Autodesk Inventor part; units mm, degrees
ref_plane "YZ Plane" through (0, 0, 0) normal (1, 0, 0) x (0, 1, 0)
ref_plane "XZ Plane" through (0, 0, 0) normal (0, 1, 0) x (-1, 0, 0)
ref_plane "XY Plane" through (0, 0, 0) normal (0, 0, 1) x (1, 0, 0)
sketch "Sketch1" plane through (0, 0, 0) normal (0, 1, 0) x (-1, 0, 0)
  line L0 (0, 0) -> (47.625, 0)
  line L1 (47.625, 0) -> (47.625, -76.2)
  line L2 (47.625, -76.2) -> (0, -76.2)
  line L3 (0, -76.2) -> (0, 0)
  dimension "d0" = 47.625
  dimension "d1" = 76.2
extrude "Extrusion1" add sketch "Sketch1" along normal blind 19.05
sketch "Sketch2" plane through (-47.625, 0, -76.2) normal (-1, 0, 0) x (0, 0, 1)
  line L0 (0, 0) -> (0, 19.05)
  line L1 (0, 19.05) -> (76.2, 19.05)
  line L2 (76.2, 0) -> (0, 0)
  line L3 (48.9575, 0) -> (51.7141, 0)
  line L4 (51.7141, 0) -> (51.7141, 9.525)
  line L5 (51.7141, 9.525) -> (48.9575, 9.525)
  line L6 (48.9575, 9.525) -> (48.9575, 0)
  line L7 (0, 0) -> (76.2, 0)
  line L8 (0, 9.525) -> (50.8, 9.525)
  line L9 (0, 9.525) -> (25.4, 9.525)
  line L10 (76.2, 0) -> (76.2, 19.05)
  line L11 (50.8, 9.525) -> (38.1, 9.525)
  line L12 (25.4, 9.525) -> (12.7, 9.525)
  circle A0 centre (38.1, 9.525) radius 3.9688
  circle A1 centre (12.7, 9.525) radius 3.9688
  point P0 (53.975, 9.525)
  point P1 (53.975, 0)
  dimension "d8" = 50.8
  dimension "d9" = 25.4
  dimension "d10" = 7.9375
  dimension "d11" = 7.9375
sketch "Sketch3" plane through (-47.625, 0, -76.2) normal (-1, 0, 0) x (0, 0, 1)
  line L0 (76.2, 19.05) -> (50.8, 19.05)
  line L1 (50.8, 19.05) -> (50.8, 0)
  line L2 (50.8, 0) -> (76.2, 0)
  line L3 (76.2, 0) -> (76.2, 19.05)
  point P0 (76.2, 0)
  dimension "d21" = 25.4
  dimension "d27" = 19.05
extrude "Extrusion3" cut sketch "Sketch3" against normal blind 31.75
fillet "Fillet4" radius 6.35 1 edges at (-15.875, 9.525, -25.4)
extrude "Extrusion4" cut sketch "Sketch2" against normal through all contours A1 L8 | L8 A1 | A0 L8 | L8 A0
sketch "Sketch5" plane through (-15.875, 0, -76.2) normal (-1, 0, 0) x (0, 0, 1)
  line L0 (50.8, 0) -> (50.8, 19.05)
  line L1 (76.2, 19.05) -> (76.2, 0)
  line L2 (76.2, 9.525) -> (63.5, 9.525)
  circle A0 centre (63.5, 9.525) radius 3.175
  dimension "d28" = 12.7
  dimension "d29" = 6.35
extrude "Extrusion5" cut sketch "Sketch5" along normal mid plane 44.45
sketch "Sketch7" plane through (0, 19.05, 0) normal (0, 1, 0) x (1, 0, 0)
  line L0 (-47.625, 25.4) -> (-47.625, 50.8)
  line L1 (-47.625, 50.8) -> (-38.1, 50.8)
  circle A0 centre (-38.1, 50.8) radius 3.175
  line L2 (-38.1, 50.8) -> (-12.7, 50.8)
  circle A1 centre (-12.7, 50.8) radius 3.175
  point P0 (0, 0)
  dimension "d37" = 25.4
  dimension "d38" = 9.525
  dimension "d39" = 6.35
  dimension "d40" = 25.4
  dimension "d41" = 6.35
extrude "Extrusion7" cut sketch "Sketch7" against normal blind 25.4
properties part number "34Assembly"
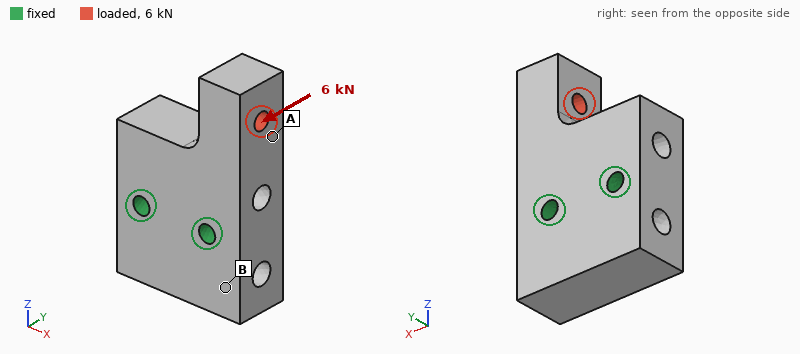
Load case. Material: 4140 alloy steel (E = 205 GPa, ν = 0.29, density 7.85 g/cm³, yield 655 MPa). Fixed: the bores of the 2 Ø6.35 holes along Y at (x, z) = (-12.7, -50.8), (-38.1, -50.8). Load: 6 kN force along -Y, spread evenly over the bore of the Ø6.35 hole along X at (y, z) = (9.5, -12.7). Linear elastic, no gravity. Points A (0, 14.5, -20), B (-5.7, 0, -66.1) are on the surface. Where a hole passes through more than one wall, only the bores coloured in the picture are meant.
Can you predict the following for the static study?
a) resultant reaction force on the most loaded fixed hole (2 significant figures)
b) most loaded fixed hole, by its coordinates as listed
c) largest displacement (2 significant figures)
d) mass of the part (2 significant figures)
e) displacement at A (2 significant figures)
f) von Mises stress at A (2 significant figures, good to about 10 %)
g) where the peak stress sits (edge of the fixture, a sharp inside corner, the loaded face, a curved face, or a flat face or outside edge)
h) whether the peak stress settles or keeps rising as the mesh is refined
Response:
5.4 kN
(-12.7, -50.8)
70 µm
370 g
36 µm
37 MPa
edge of the fixture
keeps rising
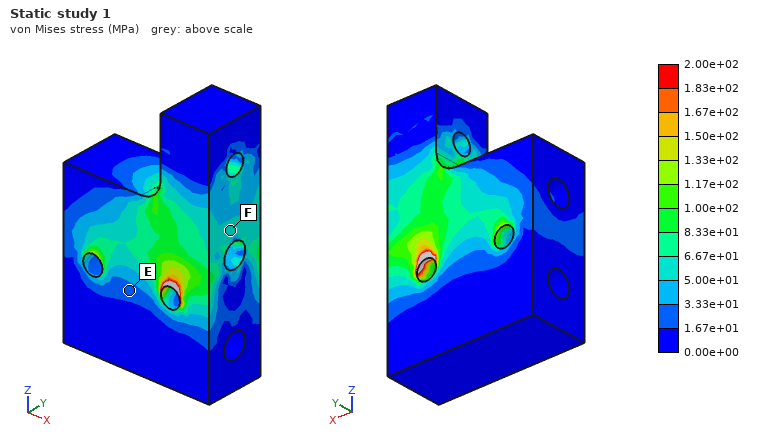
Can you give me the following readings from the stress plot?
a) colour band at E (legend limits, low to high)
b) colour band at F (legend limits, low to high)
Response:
1.67e+01 to 3.33e+01 MPa
5.00e+01 to 6.67e+01 MPa
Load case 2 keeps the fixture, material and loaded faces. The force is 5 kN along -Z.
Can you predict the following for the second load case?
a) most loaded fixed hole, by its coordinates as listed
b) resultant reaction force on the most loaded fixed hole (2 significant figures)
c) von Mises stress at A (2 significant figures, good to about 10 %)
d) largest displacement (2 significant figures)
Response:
(-12.7, -50.8)
5.5 kN
19 MPa
7.6 µm
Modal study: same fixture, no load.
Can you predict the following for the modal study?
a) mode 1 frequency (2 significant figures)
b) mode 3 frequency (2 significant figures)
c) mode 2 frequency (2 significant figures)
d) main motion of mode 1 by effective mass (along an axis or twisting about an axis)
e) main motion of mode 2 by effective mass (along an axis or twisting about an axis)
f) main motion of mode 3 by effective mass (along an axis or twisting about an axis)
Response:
6800 Hz
16 kHz
9200 Hz
along Y
along X
along Y
